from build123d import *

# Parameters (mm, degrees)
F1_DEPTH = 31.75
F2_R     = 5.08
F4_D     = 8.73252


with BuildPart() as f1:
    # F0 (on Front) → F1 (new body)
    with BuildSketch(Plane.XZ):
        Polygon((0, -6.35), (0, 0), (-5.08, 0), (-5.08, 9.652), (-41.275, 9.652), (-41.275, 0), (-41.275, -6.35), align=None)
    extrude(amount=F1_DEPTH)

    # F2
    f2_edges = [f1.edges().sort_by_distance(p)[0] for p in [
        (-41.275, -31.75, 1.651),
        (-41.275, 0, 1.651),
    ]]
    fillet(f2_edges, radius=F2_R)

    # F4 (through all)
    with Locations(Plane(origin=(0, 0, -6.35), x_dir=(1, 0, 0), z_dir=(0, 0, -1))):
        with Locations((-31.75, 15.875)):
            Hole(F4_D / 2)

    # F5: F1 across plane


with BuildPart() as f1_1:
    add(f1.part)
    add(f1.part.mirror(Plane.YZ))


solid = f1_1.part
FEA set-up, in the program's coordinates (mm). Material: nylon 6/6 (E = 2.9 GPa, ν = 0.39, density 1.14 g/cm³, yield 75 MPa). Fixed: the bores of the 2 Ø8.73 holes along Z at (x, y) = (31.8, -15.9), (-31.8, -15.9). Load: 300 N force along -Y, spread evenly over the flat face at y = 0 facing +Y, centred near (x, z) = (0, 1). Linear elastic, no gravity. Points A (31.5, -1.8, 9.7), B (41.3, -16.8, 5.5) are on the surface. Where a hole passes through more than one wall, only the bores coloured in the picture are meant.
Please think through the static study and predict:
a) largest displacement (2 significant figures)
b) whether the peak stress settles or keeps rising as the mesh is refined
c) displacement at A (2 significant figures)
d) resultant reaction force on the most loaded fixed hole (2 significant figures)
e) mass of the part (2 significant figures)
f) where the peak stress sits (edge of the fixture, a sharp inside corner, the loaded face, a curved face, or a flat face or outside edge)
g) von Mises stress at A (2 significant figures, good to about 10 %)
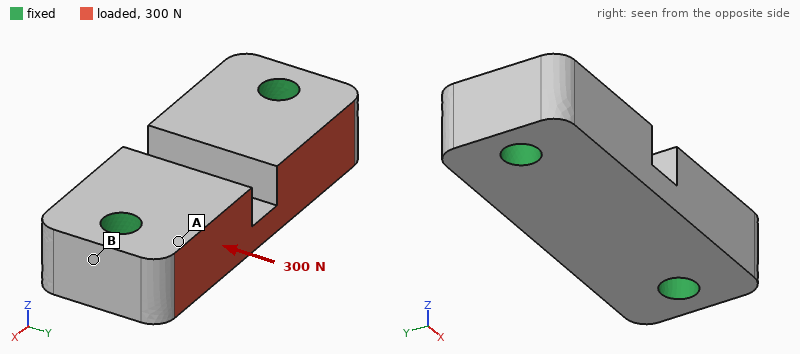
11 µm
keeps rising
3.3 µm
150 N
42 g
edge of the fixture
0.38 MPa
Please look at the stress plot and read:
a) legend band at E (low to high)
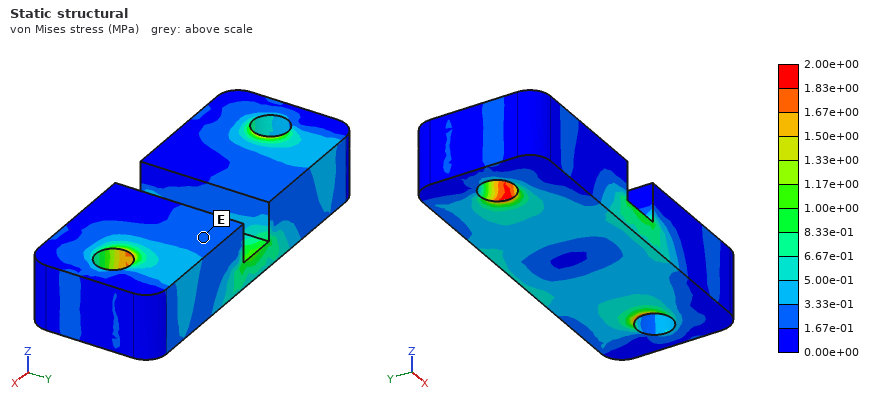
1.67e-01 to 3.33e-01 MPa
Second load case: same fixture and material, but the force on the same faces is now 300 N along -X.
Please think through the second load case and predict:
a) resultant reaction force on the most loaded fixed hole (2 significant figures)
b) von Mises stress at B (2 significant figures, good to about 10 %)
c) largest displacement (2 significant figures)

160 N
0.39 MPa
8.9 µm
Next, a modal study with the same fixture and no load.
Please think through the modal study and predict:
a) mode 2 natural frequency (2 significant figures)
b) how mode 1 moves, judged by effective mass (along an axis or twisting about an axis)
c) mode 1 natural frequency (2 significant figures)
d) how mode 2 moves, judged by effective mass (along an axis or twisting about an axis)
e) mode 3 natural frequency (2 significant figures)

5000 Hz
along Z
4700 Hz
along Y
6300 Hz
